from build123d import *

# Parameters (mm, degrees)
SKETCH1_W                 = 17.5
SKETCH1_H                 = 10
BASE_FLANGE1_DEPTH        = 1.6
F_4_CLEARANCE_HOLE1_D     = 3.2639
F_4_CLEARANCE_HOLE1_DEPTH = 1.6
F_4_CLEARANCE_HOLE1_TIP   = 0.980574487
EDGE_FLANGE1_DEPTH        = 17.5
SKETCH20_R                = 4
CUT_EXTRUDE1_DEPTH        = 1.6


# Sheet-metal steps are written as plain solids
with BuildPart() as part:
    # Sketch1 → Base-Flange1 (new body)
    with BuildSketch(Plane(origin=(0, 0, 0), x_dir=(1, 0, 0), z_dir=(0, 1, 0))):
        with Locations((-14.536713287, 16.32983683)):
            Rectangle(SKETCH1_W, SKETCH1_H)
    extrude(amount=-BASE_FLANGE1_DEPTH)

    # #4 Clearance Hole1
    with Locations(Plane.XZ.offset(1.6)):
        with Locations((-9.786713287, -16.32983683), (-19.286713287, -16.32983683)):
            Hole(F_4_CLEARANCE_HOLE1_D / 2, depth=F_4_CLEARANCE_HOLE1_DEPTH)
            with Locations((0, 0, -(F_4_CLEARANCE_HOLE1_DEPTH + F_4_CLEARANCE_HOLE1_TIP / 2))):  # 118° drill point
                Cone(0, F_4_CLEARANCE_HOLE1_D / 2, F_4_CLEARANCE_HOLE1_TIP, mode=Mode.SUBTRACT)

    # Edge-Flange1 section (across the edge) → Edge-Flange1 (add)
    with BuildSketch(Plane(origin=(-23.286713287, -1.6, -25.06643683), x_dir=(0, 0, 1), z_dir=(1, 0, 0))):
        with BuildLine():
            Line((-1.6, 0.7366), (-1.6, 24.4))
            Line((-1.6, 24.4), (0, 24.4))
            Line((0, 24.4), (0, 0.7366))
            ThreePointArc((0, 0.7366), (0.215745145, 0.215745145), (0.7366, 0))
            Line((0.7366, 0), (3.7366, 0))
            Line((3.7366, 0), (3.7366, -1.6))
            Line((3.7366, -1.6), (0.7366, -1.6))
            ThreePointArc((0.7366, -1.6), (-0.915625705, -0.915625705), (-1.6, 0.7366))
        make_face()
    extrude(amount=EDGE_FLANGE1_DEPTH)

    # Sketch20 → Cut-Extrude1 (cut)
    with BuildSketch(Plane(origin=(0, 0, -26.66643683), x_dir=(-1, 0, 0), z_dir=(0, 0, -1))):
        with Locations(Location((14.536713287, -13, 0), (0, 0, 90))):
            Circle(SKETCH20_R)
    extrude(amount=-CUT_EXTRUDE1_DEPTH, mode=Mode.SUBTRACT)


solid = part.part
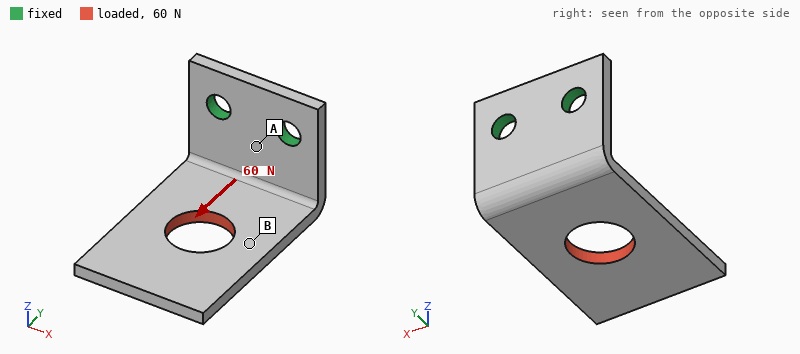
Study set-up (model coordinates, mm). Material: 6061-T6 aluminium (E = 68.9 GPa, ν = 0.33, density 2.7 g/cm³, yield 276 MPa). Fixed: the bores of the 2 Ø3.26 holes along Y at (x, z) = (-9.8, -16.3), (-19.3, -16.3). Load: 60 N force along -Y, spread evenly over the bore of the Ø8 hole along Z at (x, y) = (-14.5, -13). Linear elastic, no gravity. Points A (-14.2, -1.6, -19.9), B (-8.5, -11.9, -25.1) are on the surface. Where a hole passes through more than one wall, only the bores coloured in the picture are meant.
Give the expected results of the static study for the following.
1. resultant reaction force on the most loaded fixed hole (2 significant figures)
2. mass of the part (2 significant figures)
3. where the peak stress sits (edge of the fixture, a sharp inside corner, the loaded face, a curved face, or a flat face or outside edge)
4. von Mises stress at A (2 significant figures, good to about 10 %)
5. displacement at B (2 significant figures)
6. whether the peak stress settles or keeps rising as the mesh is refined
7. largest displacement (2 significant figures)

30 N
2.7 g
edge of the fixture
38 MPa
0.061 mm
keeps rising
0.13 mm
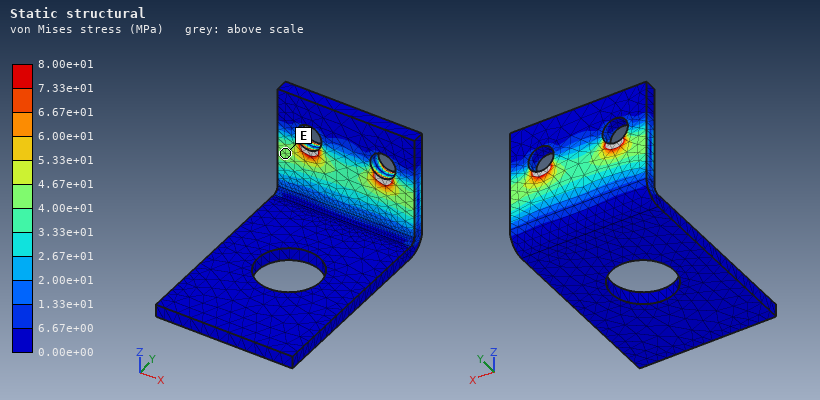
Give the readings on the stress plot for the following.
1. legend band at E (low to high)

4.00e+01 to 4.67e+01 MPa
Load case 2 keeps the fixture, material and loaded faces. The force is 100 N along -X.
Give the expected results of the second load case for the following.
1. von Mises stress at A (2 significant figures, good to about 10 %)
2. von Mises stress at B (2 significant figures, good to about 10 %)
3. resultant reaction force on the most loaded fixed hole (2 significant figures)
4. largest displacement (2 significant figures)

62 MPa
18 MPa
140 N
0.20 mm
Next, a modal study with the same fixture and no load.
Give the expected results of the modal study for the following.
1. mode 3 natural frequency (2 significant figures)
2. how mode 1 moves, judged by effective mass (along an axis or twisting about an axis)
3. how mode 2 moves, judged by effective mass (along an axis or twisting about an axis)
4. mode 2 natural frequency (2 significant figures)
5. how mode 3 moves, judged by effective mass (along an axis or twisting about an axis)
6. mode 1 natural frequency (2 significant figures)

5800 Hz
along Z
along X
3100 Hz
twisting about Y
1400 Hz
